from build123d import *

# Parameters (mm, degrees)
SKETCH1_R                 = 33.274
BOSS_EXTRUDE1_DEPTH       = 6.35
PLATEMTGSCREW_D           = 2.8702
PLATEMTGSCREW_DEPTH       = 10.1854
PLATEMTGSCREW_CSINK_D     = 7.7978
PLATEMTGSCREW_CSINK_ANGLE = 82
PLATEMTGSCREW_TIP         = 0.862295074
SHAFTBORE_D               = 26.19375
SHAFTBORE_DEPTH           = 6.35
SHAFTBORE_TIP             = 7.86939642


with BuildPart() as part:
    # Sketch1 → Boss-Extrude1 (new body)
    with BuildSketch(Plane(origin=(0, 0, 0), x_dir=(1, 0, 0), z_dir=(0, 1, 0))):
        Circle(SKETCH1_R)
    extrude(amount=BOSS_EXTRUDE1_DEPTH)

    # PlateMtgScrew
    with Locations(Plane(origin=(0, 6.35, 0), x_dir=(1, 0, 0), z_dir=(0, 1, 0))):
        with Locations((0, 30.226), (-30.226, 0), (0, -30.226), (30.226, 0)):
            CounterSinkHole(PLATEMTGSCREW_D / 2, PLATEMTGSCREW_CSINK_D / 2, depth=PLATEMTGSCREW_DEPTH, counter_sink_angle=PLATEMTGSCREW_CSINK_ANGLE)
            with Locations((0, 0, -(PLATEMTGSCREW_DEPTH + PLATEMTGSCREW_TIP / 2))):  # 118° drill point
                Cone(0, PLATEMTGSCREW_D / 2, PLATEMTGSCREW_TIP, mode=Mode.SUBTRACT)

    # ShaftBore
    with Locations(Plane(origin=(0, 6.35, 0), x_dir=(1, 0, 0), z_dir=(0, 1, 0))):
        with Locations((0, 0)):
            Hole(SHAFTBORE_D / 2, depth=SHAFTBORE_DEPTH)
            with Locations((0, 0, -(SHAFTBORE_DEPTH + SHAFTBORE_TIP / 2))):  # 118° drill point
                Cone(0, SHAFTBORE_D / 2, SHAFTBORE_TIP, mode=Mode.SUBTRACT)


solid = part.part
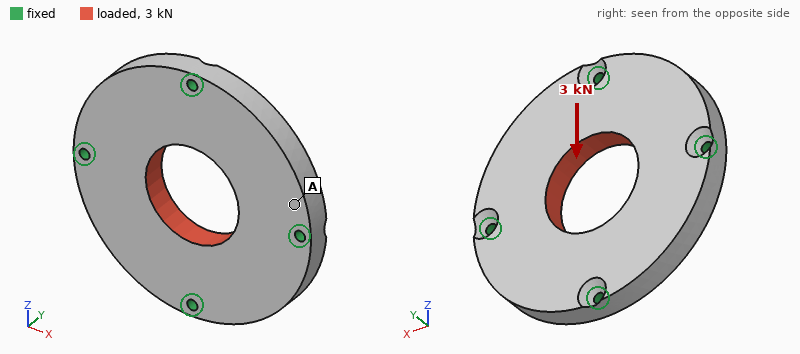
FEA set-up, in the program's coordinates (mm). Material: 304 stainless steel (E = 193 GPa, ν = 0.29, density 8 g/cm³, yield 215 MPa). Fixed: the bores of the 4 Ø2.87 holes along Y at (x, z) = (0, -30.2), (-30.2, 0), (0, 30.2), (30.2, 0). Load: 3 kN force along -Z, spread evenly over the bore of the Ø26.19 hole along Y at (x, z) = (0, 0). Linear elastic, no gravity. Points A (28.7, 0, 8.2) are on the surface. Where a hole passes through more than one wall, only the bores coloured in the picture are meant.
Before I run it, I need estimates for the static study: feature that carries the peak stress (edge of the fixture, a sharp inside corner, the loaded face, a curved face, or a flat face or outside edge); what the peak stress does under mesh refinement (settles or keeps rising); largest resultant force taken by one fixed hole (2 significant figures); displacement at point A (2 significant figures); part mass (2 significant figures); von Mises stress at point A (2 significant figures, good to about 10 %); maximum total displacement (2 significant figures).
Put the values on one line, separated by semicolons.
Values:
edge of the fixture; keeps rising; 840 N; 0.51 µm; 150 g; 8.3 MPa; 1.5 µm
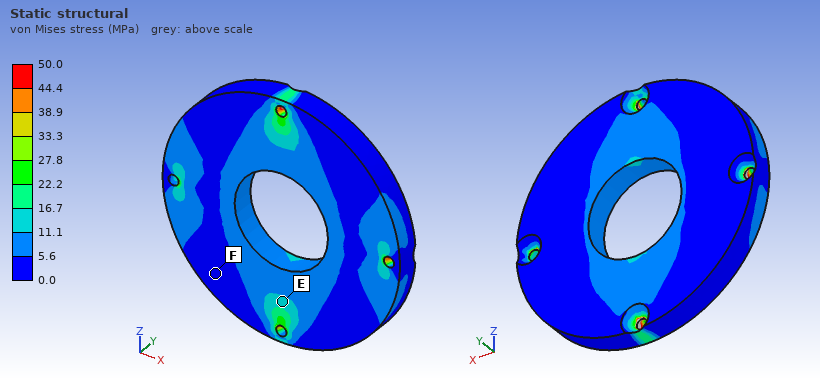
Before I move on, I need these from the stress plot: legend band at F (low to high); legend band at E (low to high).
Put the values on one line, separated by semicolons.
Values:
0.0 to 5.6 MPa; 11.1 to 16.7 MPa
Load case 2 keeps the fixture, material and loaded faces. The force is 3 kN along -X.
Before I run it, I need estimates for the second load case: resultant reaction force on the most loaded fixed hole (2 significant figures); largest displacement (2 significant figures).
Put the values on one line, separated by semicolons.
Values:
840 N; 1.5 µm
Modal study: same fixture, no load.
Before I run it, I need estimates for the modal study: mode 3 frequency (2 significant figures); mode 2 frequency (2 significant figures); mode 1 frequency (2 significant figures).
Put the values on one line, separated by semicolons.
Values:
11 kHz; 9900 Hz; 9500 Hz
